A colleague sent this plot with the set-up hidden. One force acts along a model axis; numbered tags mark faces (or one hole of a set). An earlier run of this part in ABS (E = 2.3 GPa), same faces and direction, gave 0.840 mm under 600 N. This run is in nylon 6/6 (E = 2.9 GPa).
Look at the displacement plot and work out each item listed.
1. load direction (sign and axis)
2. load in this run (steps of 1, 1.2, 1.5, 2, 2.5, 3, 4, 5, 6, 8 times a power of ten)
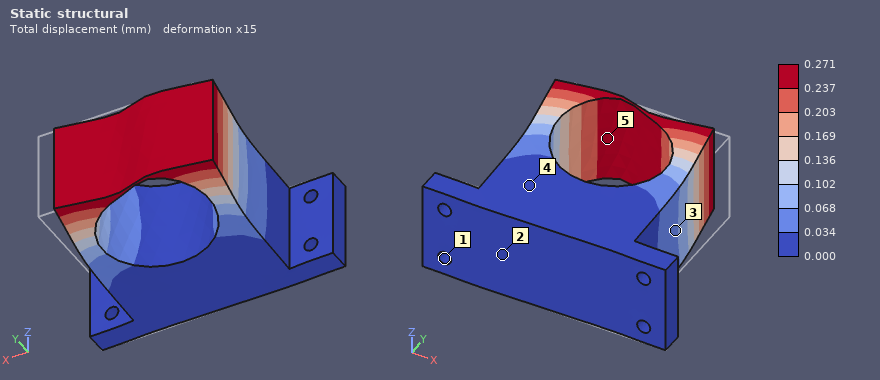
-X
250 N
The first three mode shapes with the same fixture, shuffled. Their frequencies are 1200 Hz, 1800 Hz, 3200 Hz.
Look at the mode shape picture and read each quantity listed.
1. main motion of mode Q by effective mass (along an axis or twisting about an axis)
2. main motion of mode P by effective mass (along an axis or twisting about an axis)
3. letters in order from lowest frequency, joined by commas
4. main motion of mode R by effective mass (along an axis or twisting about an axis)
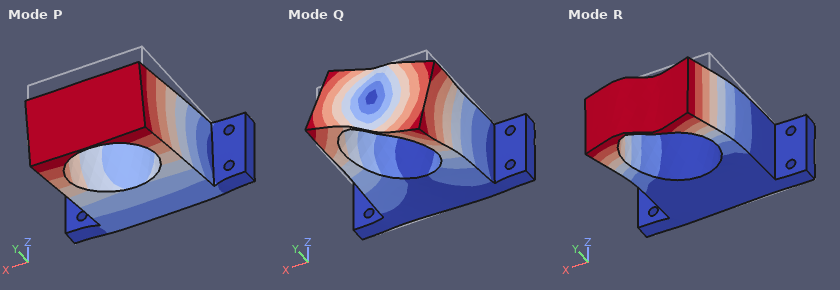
twisting about Y
along Z
P, R, Q
along X
